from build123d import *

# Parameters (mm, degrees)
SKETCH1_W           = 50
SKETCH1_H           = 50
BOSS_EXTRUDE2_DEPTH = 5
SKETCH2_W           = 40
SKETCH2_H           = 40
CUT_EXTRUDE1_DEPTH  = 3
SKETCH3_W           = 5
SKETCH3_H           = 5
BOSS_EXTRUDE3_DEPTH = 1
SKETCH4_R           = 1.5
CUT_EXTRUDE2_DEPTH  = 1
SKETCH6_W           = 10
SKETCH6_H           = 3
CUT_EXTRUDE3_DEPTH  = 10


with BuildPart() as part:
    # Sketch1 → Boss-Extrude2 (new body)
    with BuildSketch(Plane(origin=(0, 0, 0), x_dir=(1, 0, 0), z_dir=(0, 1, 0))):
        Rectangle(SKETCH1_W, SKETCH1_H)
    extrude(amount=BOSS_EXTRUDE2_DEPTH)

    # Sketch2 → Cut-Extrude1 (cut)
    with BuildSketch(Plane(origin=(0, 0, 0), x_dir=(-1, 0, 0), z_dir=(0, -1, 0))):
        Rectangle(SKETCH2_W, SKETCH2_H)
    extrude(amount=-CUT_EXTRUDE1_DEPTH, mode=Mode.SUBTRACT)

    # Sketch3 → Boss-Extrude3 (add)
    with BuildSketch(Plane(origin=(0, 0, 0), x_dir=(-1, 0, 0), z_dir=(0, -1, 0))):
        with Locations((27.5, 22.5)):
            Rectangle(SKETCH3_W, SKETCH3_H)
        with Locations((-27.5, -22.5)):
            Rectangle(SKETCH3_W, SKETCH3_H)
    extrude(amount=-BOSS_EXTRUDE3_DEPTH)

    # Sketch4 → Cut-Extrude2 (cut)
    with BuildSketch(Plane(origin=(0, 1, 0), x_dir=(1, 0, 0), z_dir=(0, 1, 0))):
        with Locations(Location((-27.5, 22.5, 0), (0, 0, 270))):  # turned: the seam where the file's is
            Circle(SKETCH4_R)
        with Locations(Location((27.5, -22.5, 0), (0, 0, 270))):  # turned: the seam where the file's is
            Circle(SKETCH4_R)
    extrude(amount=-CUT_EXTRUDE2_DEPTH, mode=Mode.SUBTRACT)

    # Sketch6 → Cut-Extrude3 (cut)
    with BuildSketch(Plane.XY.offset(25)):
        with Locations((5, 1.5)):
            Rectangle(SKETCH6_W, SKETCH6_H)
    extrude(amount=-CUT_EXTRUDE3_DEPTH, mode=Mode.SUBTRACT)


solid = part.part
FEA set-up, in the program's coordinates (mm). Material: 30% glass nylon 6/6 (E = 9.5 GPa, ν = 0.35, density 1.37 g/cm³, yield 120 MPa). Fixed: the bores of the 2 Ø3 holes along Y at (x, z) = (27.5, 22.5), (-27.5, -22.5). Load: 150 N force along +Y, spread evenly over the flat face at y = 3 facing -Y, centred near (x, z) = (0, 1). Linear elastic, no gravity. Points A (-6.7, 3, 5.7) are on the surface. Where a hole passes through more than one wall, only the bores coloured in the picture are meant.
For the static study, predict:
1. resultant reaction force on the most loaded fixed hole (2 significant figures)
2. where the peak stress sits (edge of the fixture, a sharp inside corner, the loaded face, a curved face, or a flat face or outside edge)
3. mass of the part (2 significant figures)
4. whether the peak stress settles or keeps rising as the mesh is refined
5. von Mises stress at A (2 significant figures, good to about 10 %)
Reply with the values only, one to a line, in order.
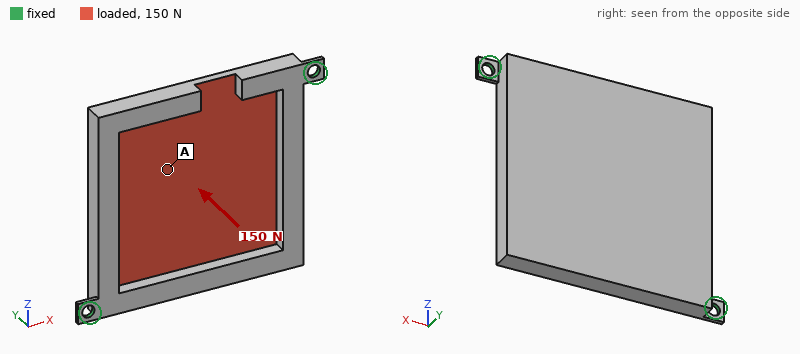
290 N
edge of the fixture
10 g
keeps rising
6.7 MPa
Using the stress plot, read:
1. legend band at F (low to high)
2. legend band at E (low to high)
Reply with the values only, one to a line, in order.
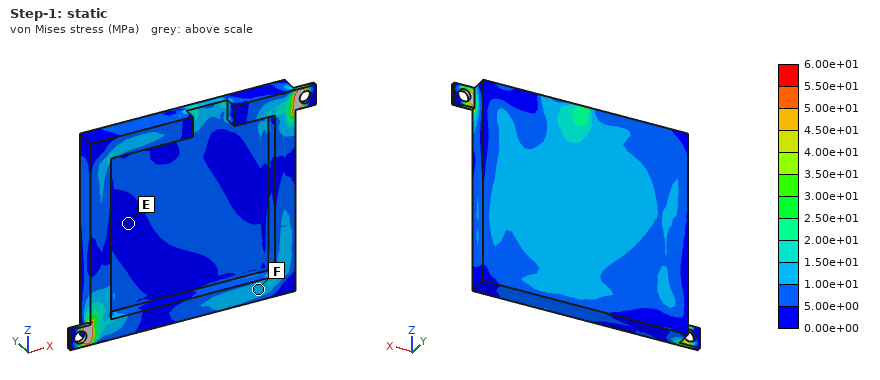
1.00e+01 to 1.50e+01 MPa
0.00e+00 to 5.00e+00 MPa
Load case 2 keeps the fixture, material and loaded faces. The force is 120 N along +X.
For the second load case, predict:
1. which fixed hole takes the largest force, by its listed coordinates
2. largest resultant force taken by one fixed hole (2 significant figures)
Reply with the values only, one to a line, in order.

(-27.5, -22.5)
65 N
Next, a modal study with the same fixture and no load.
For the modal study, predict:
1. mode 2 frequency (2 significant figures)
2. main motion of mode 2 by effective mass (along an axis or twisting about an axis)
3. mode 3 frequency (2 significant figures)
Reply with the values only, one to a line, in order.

1000 Hz
along Y
2100 Hz
